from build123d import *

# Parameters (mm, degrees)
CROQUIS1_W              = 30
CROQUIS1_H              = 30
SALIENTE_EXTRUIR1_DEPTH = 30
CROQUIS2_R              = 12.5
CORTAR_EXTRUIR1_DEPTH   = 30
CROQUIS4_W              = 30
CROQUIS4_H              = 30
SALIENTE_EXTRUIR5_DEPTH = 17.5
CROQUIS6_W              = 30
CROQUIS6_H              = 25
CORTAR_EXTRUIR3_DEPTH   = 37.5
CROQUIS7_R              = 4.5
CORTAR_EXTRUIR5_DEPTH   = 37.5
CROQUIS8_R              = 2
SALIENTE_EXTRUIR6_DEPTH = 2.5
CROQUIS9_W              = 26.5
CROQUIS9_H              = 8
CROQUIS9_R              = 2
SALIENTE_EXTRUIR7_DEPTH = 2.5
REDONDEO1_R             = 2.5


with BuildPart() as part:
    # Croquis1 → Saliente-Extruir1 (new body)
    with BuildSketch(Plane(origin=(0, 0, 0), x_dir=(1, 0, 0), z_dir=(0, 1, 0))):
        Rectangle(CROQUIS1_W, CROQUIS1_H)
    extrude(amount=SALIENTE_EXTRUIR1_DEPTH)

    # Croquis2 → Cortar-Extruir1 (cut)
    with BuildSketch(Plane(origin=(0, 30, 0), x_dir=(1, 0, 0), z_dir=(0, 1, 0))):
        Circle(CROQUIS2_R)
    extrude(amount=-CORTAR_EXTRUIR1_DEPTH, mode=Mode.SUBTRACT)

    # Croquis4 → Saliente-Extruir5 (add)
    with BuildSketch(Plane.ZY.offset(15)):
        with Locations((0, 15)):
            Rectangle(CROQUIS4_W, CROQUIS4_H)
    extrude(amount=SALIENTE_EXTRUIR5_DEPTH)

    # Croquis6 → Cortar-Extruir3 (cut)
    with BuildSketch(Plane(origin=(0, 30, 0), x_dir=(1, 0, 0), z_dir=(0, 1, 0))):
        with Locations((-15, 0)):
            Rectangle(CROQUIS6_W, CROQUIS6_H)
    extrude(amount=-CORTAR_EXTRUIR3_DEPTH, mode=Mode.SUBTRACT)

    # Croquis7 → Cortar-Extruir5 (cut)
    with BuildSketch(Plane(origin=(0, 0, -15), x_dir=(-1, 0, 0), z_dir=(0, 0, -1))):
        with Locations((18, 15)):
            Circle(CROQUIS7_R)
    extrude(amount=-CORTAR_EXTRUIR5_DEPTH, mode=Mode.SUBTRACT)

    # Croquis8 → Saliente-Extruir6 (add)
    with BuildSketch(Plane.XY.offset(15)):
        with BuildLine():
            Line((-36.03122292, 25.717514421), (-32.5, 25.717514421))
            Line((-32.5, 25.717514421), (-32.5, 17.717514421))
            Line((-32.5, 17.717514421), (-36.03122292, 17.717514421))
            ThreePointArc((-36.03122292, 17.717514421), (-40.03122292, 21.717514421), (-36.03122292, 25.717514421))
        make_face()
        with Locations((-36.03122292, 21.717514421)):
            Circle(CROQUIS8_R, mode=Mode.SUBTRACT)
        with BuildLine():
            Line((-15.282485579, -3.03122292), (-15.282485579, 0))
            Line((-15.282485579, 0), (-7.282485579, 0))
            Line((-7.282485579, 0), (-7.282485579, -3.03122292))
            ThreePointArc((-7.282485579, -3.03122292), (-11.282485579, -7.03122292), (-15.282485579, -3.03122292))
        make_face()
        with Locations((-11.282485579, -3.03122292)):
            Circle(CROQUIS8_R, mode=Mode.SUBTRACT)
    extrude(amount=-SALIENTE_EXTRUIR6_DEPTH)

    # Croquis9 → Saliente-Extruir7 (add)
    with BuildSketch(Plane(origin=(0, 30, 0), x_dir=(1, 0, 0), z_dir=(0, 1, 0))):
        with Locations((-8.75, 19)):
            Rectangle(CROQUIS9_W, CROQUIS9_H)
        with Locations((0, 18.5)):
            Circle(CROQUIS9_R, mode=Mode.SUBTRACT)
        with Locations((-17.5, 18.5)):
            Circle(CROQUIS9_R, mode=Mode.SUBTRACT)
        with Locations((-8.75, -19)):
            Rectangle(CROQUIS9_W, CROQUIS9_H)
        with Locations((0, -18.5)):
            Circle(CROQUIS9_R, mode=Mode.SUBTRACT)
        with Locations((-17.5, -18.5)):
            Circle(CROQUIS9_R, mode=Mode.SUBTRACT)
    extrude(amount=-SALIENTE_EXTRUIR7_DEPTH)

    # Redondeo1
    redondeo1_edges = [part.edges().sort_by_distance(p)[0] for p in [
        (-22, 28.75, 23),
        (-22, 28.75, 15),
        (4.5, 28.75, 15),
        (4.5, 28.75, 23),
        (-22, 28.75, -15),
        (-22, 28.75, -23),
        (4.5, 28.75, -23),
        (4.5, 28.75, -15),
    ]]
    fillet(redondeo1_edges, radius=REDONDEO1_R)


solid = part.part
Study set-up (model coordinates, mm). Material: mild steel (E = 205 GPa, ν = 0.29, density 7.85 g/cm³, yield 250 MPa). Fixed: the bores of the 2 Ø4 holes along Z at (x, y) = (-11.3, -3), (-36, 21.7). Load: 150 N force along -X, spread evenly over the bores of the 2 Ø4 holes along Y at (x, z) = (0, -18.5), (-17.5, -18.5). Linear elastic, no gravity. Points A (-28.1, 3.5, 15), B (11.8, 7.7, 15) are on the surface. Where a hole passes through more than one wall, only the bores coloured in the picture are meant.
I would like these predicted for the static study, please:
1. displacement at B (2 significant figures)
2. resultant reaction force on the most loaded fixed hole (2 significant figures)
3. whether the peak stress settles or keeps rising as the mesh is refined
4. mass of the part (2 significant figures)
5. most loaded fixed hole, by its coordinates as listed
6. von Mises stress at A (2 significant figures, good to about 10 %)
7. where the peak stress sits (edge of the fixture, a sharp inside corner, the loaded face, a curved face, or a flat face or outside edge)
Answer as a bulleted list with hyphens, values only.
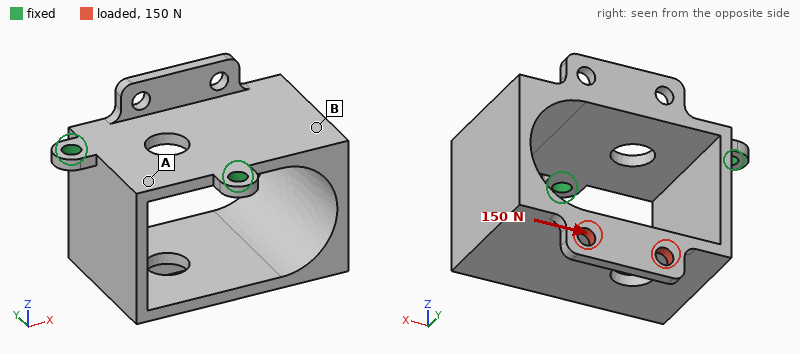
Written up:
- 0.078 mm
- 210 N
- keeps rising
- 110 g
- (-36, 21.7)
- 24 MPa
- edge of the fixture
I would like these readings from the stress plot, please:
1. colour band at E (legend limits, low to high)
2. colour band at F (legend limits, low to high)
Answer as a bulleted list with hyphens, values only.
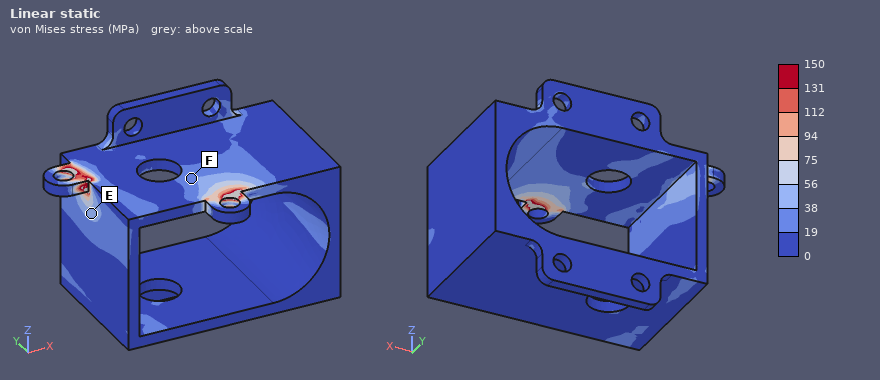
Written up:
- 38 to 56 MPa
- 19 to 38 MPa
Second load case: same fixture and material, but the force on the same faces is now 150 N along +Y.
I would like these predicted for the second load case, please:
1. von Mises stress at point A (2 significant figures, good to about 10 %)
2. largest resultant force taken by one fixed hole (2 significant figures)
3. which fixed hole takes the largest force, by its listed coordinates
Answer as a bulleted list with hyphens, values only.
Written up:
- 27 MPa
- 130 N
- (-11.3, -3)
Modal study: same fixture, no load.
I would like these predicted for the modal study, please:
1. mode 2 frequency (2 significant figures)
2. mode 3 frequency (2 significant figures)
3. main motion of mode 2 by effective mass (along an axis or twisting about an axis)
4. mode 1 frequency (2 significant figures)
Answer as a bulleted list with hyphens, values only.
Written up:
- 1400 Hz
- 2600 Hz
- along Y
- 600 Hz
